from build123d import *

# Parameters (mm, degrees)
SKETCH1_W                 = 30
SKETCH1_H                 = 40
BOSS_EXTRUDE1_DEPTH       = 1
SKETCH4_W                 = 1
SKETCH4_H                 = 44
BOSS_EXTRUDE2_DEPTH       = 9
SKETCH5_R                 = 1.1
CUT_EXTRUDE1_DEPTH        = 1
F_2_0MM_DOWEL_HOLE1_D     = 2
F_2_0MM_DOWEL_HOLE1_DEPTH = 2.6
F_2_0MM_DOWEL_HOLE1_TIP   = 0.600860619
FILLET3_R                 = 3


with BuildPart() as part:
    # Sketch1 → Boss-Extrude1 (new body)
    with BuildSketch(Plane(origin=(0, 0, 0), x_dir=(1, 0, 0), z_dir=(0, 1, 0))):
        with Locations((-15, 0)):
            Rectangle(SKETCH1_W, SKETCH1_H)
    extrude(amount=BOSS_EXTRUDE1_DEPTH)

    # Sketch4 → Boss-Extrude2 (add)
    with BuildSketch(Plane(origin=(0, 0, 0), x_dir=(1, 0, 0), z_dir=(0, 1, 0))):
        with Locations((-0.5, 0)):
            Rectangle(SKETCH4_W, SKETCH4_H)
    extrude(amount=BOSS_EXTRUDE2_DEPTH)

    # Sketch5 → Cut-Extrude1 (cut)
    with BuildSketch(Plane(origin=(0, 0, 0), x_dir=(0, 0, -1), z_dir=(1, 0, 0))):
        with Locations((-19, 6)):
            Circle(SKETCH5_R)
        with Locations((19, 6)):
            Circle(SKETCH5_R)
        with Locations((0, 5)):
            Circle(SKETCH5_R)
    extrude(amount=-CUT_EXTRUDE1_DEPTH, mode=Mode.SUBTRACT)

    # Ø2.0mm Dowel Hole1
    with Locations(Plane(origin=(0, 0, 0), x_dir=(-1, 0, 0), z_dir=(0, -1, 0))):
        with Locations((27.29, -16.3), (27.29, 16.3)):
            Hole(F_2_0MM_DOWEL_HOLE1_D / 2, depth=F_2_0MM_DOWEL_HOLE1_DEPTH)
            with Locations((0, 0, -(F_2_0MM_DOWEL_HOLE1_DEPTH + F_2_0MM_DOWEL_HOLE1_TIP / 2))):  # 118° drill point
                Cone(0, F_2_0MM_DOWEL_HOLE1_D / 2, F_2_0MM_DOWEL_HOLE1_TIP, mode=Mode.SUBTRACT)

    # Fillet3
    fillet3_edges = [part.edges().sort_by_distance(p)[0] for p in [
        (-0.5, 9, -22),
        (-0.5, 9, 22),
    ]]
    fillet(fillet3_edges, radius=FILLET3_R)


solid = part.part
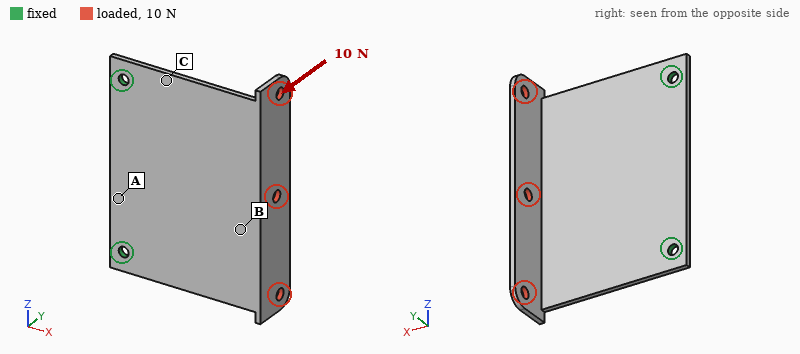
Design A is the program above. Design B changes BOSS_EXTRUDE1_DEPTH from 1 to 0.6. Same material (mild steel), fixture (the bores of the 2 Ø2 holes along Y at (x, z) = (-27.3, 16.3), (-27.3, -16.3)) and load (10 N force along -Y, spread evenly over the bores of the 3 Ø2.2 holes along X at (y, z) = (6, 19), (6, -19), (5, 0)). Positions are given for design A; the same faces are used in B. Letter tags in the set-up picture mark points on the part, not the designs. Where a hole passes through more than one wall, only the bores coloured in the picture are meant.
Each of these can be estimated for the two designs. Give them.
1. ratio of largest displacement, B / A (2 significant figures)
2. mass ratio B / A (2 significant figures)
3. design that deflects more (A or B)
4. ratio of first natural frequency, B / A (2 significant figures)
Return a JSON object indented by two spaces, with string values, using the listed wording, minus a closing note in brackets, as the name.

{
  "ratio of largest displacement, B / A": "4.5",
  "mass ratio B / A": "0.70",
  "design that deflects more": "B",
  "ratio of first natural frequency, B / A": "0.51"
}
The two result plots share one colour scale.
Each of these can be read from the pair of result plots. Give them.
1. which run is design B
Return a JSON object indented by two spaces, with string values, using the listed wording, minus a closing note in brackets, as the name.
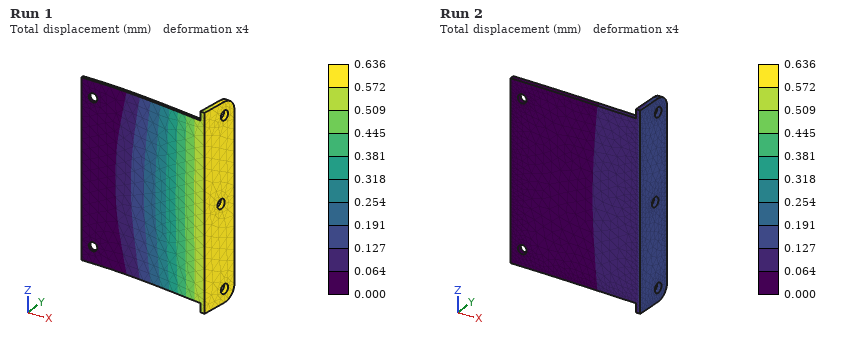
{
  "which run is design B": "Run 1"
}
